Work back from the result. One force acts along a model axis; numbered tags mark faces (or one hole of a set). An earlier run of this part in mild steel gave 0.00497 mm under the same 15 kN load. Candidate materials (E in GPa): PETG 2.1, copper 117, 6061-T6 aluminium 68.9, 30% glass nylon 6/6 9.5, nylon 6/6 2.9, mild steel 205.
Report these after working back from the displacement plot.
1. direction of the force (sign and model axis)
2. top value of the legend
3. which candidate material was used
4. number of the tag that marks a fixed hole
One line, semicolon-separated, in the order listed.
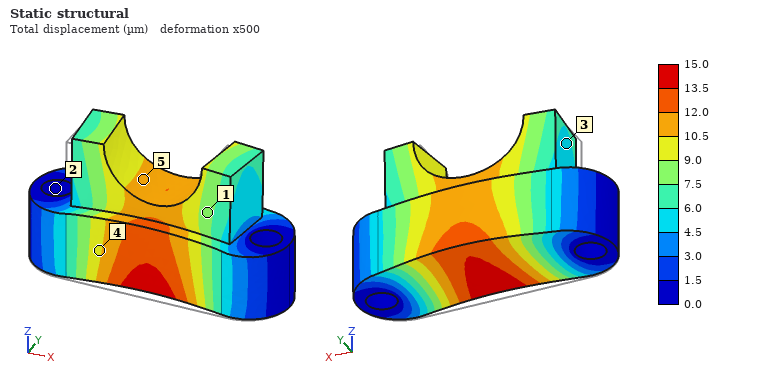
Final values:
+Y; 15.0 µm; 6061-T6 aluminium; 2
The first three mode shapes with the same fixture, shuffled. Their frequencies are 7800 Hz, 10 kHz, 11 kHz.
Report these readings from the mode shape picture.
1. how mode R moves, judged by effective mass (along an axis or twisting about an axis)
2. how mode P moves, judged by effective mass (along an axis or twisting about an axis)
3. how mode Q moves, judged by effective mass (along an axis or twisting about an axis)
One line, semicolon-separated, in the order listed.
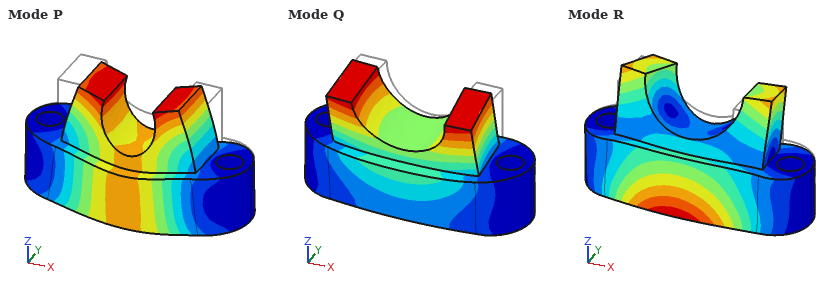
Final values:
along Y; along Z; along Y
